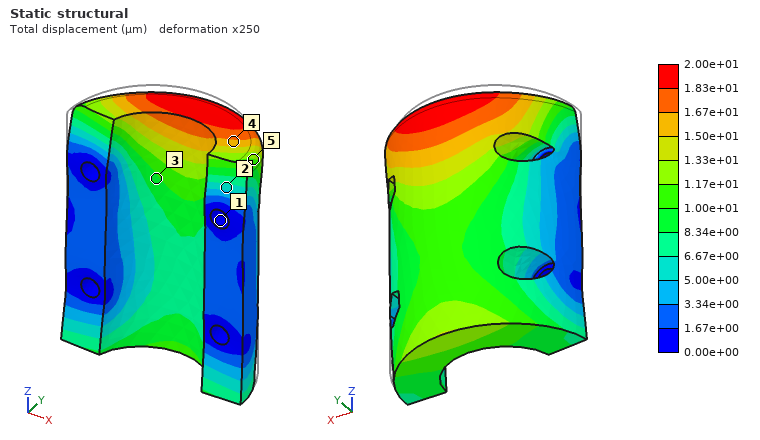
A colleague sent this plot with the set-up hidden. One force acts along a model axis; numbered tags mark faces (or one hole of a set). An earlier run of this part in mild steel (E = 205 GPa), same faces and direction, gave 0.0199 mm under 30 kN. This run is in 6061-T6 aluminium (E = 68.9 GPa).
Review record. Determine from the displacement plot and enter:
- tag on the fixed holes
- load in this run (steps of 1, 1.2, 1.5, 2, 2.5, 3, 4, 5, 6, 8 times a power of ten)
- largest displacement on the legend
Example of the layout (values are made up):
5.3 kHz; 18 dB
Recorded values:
1; 10 kN; 2.00e+01 µm
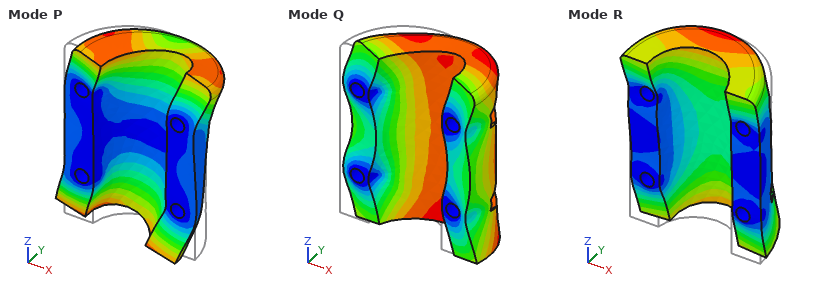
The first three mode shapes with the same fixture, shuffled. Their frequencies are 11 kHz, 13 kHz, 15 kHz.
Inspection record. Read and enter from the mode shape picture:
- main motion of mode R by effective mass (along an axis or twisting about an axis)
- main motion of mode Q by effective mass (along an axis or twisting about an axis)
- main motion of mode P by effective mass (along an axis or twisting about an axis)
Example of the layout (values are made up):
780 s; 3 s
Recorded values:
along Z; along X; twisting about Y
